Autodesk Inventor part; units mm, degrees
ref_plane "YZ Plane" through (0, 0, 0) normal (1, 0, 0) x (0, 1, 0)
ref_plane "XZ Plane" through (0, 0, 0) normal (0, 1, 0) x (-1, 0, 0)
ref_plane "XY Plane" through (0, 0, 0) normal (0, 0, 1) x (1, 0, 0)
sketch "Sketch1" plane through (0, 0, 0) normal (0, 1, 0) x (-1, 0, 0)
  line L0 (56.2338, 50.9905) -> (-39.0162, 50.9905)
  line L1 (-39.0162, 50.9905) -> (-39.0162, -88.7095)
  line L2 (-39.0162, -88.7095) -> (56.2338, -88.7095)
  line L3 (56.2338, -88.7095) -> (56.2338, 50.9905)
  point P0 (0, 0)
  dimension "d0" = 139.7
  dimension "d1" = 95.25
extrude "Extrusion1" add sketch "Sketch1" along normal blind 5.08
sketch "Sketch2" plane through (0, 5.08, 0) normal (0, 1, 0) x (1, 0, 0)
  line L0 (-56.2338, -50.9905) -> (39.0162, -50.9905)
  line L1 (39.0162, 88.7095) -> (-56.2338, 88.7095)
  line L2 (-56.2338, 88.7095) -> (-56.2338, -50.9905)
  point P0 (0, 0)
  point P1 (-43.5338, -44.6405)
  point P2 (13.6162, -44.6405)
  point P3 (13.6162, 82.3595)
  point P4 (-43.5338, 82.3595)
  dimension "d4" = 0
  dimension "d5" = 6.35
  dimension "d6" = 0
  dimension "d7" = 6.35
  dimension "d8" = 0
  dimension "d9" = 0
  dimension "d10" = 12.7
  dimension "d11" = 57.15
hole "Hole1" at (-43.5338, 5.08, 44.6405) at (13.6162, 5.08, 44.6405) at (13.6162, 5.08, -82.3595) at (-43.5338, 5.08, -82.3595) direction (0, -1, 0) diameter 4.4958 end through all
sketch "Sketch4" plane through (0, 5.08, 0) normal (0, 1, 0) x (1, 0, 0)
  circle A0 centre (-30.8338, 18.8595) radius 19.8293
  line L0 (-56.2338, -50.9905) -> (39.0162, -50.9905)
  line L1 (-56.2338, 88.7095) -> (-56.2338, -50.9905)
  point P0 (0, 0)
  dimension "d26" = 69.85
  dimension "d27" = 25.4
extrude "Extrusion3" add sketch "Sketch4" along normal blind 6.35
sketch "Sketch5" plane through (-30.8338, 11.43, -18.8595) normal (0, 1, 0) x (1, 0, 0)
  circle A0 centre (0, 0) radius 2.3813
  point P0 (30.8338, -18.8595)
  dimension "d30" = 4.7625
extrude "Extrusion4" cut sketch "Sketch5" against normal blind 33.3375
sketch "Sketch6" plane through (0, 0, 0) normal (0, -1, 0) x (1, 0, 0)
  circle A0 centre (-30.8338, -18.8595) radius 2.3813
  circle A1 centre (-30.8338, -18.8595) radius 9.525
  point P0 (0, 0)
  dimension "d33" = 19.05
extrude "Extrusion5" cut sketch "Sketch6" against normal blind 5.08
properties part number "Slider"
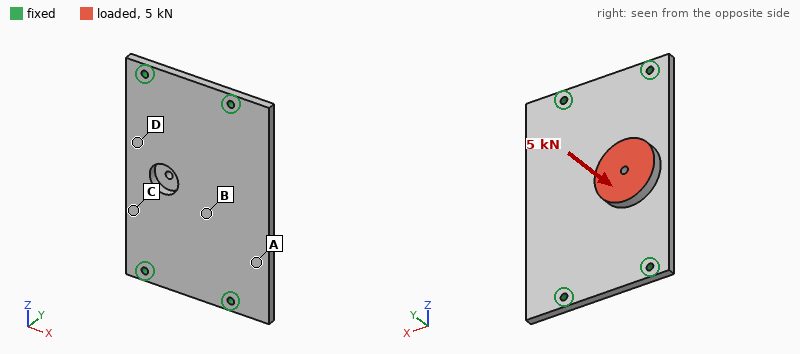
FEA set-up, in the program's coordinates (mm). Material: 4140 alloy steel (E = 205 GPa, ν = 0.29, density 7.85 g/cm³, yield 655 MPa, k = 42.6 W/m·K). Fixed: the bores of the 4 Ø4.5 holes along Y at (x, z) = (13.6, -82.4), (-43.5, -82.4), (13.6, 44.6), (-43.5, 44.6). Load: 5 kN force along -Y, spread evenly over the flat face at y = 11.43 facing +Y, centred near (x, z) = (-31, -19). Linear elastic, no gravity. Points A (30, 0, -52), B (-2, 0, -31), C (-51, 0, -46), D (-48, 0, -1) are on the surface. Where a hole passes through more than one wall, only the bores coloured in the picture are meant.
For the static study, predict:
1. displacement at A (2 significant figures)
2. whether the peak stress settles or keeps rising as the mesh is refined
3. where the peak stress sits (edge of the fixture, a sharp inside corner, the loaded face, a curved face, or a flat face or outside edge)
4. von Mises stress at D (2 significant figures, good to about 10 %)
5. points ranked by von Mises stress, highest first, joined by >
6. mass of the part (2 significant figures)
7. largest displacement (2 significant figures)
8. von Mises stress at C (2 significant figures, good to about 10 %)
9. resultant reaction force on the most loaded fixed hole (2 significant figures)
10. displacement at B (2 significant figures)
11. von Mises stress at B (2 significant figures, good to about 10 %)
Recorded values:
0.047 mm
keeps rising
edge of the fixture
170 MPa
D > C > B > A
580 g
0.31 mm
130 MPa
2.6 kN
0.17 mm
73 MPa
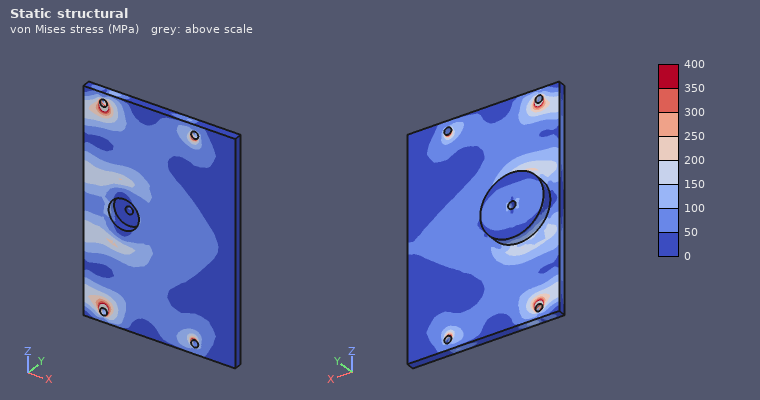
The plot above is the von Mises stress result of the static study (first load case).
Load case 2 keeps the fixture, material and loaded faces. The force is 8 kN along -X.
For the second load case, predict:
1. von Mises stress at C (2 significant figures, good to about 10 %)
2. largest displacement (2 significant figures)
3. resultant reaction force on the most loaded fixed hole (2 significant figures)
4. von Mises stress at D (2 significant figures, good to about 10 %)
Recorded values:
57 MPa
0.14 mm
2.6 kN
75 MPa
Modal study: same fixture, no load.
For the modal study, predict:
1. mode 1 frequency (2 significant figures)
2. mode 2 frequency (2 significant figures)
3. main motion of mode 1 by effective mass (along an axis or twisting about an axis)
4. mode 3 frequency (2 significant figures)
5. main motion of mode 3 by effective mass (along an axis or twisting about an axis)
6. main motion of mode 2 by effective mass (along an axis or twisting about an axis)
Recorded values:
1400 Hz
1900 Hz
along Y
3800 Hz
twisting about X
twisting about Z
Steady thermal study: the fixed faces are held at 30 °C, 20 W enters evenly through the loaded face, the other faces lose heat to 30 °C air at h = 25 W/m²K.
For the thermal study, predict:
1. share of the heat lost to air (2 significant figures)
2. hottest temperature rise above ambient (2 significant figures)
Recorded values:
43 %
33 K
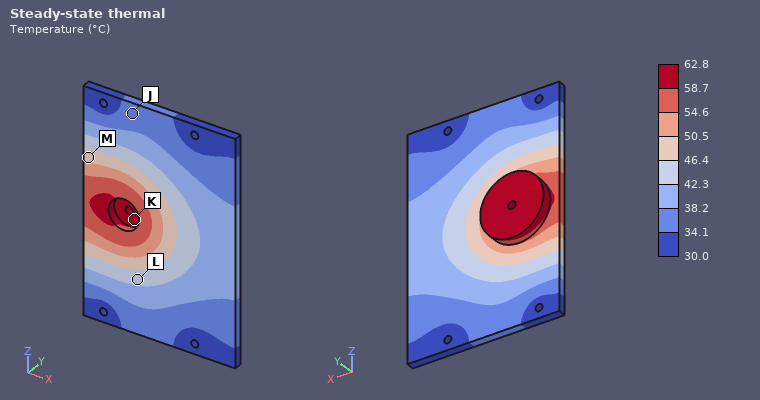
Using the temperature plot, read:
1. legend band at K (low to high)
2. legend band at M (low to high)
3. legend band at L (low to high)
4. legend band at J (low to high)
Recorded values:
58.7 to 62.8 °C
46.4 to 50.5 °C
42.3 to 46.4 °C
34.1 to 38.2 °C
